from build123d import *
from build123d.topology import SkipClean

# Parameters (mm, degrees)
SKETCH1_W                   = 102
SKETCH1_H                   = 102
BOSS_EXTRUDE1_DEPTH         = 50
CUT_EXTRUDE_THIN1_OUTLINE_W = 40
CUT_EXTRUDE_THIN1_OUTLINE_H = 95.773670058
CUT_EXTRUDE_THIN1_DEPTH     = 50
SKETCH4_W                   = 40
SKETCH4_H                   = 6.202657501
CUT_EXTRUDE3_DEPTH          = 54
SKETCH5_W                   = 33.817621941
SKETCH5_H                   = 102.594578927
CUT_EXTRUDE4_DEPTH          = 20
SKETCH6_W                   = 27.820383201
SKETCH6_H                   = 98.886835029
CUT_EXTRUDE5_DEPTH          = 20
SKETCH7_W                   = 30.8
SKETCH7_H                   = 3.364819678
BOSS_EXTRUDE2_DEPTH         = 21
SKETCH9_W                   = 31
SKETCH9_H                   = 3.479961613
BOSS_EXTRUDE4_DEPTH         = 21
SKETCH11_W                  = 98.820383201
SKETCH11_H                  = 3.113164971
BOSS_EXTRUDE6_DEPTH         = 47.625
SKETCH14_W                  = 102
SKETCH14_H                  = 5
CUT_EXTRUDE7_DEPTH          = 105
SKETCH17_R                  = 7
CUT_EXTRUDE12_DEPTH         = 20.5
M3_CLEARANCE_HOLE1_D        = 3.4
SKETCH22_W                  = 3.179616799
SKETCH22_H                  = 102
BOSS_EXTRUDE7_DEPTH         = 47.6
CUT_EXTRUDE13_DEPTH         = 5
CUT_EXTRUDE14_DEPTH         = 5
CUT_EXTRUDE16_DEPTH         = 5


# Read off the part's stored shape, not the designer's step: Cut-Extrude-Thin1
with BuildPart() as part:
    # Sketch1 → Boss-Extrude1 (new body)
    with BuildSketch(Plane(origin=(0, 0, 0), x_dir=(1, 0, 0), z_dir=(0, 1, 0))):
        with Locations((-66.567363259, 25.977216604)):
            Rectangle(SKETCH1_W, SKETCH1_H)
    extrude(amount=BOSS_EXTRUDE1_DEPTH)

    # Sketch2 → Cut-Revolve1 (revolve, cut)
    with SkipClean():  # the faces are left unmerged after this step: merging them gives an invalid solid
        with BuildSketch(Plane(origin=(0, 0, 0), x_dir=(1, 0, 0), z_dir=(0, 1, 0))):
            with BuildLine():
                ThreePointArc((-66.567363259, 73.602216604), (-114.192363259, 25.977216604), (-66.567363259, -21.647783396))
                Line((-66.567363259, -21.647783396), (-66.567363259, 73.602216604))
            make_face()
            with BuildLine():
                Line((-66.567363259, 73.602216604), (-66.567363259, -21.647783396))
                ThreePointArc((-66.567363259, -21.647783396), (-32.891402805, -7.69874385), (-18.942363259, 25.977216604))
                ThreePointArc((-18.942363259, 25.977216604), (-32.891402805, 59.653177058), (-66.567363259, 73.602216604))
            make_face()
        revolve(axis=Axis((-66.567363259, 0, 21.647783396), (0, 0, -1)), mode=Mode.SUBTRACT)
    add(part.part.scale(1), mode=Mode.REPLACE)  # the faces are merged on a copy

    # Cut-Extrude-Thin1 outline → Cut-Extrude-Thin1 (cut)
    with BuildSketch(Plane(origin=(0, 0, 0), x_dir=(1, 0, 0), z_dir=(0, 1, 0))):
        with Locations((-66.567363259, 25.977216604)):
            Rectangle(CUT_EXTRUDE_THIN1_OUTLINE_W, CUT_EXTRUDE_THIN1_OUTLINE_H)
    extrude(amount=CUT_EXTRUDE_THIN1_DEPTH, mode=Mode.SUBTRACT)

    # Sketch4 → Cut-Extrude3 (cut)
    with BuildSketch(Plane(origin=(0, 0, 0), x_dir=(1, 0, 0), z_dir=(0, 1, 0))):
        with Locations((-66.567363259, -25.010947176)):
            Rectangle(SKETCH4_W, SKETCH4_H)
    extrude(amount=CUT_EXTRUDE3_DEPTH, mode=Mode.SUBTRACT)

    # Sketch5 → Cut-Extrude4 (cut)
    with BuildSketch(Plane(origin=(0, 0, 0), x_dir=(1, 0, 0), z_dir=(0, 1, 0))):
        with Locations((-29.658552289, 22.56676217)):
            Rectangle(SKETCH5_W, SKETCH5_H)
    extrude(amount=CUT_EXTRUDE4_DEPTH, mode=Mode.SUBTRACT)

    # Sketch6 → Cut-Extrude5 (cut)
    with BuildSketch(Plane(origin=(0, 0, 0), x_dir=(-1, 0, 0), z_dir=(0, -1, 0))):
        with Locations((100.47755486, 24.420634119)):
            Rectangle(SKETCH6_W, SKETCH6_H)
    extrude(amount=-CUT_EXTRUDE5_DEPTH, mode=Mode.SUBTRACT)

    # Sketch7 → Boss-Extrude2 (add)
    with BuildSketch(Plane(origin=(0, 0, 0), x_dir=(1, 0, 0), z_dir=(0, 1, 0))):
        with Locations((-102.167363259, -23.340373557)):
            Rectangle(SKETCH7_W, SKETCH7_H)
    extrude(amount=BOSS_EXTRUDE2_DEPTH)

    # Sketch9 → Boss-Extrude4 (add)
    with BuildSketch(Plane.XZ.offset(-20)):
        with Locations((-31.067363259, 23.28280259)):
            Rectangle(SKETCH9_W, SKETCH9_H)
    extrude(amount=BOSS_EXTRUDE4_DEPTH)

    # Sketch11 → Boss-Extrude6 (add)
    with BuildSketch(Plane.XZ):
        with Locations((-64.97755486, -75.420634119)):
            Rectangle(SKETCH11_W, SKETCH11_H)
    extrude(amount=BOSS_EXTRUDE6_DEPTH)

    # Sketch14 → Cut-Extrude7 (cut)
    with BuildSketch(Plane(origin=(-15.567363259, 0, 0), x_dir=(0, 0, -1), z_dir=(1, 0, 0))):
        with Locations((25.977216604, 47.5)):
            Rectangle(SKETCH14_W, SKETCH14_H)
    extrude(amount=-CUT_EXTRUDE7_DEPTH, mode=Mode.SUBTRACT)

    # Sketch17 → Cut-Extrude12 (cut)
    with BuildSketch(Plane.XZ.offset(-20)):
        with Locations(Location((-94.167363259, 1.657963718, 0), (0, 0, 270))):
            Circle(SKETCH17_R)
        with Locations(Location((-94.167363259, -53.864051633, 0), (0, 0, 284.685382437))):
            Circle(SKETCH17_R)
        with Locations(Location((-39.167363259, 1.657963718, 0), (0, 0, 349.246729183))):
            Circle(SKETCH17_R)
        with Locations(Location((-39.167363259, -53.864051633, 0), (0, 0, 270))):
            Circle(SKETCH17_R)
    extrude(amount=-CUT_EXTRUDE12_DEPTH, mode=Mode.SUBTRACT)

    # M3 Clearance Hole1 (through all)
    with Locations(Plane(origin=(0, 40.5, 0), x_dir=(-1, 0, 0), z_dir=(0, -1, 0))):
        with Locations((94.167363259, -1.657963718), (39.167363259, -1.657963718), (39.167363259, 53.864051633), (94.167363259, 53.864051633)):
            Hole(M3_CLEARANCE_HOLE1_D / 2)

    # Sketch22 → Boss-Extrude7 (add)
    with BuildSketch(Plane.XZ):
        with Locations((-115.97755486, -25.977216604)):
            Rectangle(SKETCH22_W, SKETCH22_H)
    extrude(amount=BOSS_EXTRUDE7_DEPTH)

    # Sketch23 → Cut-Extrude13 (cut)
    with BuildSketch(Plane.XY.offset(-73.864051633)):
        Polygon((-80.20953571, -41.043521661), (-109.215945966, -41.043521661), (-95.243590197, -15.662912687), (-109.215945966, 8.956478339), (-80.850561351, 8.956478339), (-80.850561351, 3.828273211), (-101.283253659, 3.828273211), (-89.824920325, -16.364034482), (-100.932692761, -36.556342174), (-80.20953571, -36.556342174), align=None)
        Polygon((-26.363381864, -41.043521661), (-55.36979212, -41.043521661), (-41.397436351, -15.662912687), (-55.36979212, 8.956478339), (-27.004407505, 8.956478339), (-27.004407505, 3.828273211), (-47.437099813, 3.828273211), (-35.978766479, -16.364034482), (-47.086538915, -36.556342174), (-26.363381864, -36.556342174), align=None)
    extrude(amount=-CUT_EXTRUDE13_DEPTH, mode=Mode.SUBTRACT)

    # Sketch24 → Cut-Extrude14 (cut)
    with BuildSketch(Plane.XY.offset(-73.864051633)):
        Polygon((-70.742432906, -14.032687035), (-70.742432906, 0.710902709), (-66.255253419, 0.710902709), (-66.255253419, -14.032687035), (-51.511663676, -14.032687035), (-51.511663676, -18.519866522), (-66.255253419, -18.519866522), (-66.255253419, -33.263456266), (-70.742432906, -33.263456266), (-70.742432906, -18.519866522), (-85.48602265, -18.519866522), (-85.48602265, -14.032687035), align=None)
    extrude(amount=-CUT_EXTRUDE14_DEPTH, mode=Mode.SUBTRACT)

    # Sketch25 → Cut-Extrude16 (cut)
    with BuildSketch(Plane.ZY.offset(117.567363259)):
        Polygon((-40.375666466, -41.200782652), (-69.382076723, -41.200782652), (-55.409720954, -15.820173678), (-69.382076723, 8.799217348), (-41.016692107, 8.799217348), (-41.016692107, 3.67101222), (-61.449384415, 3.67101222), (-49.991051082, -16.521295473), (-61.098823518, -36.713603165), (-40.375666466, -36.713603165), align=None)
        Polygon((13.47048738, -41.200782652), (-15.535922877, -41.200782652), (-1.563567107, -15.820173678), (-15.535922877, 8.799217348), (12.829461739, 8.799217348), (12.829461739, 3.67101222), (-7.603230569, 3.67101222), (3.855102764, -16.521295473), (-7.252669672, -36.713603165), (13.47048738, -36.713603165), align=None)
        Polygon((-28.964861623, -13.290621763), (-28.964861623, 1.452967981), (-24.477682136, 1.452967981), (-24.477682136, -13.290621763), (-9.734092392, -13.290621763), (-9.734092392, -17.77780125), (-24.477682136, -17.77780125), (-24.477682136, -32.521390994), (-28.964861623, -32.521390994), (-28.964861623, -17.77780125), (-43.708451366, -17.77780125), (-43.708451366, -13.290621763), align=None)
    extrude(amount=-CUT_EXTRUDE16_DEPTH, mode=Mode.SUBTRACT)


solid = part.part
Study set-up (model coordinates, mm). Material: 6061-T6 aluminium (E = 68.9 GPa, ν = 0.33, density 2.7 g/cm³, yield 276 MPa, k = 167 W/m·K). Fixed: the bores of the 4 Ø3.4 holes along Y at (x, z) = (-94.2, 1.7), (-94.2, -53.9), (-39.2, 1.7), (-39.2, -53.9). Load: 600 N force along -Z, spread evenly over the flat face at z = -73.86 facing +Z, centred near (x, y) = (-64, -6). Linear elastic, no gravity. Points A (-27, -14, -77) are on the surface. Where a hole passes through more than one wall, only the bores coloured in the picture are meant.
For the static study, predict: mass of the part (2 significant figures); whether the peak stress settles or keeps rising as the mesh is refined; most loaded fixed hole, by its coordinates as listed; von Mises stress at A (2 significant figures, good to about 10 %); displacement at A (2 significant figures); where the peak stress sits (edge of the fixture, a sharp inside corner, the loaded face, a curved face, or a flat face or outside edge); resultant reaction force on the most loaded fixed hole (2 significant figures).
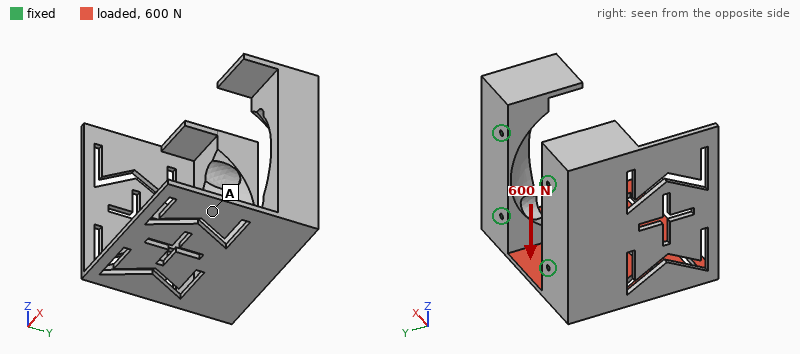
440 g
keeps rising
(-94.2, -53.9)
18 MPa
0.63 mm
a sharp inside corner
400 N
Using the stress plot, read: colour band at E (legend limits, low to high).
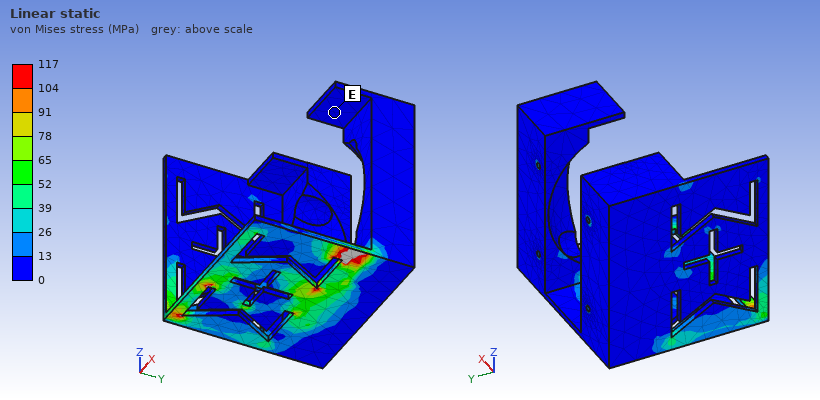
0 to 13 MPa
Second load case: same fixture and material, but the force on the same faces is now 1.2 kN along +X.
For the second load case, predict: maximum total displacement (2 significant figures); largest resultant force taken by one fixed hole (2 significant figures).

0.25 mm
1.4 kN
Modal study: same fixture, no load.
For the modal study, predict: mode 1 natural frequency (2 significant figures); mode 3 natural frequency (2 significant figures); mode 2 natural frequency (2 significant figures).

560 Hz
1200 Hz
730 Hz
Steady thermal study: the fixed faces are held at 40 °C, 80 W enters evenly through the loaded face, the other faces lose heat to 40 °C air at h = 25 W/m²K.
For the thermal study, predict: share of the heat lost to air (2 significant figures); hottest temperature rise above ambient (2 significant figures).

27 %
86 K
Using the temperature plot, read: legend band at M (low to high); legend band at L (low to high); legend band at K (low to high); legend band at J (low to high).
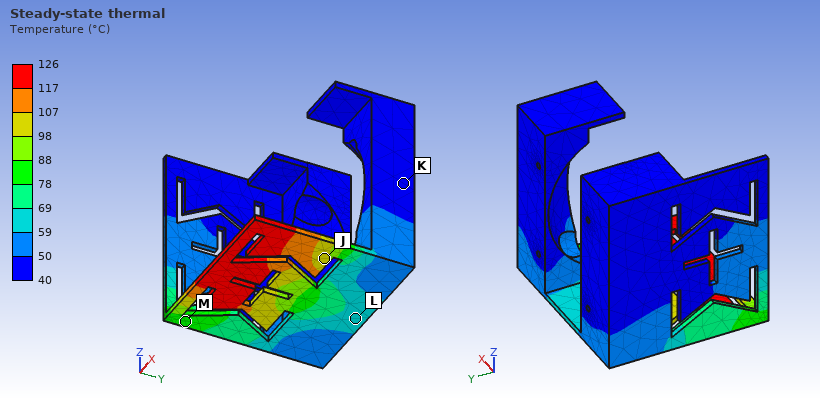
78 to 88 °C
59 to 69 °C
40 to 50 °C
98 to 107 °C
